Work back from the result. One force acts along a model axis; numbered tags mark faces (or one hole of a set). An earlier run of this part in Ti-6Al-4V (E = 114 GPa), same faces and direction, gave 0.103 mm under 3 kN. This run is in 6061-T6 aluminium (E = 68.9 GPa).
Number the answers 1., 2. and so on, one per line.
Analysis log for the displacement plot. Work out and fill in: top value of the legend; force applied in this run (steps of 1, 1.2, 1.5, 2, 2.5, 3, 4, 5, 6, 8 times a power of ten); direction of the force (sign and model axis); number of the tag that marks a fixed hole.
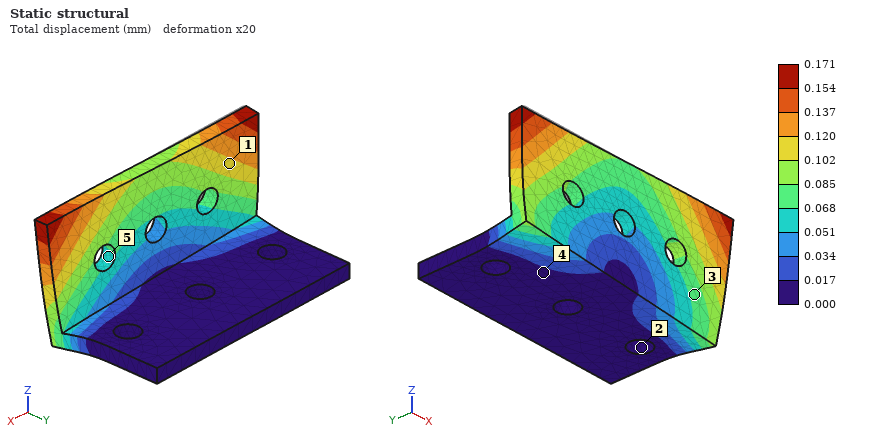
1. 0.171 mm
2. 3 kN
3. +X
4. 2
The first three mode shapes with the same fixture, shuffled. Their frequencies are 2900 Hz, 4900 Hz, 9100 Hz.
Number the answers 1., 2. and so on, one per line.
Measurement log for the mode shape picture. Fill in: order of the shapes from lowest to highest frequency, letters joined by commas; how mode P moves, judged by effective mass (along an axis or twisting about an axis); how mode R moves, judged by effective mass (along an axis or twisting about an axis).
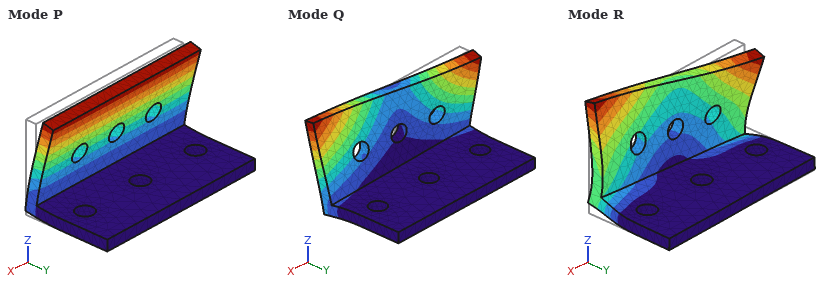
1. P, Q, R
2. along Y
3. along X
